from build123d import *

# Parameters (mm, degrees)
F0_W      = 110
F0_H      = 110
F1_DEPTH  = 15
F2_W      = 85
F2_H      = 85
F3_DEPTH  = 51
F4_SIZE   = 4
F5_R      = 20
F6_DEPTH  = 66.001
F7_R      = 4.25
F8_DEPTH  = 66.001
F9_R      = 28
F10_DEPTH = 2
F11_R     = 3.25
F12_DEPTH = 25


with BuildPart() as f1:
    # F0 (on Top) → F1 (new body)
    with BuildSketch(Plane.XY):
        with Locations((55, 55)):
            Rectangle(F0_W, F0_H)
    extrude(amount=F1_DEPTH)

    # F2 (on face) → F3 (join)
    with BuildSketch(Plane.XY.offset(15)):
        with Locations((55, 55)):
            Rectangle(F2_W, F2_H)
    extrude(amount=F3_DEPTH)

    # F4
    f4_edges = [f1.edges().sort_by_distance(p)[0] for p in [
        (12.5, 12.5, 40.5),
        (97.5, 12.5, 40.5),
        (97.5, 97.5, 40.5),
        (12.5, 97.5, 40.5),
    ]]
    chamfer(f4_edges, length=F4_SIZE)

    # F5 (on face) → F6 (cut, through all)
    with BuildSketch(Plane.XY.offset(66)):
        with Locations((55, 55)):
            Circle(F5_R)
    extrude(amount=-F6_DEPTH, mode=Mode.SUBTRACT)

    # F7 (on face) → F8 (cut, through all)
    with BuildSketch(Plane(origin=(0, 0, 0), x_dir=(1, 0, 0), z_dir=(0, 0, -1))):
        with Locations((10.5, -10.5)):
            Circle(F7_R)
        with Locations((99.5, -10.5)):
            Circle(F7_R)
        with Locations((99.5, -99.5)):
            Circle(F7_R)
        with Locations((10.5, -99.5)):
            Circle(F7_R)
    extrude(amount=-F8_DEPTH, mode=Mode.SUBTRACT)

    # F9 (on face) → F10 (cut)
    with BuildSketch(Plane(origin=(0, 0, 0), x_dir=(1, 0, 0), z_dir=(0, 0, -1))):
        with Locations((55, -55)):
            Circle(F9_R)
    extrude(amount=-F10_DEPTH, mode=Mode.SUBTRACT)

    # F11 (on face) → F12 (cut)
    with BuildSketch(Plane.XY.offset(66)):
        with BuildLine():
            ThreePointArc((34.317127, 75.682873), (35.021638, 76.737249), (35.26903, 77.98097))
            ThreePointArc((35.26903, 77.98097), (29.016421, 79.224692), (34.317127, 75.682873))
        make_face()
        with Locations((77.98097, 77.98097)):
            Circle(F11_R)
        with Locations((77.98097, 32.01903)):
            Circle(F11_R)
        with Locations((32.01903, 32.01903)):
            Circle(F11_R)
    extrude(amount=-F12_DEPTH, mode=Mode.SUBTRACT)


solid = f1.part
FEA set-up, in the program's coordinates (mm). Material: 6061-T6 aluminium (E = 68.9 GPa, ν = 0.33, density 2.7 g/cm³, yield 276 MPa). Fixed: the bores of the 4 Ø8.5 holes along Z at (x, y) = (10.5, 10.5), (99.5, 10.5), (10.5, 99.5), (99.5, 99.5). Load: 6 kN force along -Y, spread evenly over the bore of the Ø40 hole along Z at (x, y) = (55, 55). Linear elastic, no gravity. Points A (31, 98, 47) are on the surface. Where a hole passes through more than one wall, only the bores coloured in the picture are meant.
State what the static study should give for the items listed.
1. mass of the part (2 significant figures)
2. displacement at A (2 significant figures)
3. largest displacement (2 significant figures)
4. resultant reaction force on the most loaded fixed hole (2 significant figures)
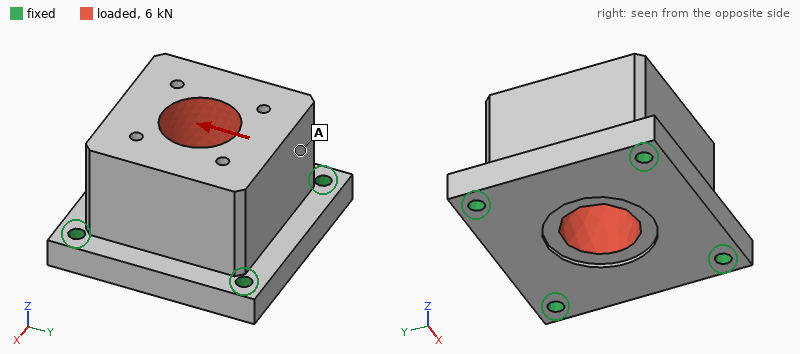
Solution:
1.2 kg
4.2 µm
5.5 µm
1.9 kN
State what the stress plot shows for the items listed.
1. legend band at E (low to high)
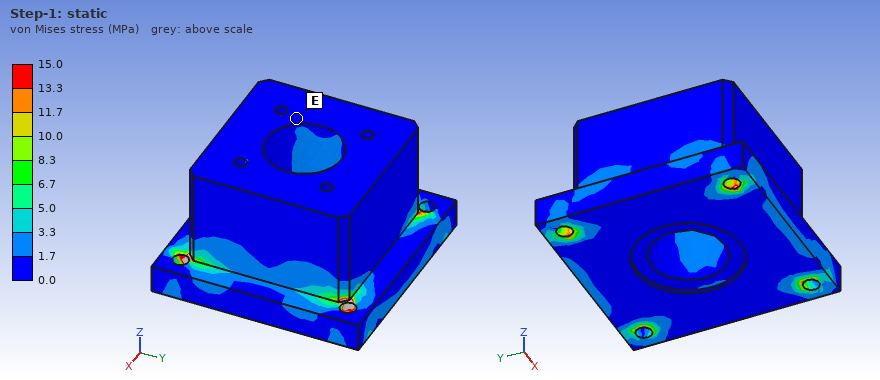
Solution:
0.0 to 1.7 MPa
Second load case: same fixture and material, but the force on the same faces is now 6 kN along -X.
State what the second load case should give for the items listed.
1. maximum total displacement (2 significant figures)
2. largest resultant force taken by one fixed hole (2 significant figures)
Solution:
5.5 µm
1.9 kN
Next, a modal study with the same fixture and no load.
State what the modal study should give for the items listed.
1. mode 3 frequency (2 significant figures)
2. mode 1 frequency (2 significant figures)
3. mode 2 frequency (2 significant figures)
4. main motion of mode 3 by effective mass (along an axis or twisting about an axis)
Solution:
6300 Hz
6000 Hz
6000 Hz
along Z
